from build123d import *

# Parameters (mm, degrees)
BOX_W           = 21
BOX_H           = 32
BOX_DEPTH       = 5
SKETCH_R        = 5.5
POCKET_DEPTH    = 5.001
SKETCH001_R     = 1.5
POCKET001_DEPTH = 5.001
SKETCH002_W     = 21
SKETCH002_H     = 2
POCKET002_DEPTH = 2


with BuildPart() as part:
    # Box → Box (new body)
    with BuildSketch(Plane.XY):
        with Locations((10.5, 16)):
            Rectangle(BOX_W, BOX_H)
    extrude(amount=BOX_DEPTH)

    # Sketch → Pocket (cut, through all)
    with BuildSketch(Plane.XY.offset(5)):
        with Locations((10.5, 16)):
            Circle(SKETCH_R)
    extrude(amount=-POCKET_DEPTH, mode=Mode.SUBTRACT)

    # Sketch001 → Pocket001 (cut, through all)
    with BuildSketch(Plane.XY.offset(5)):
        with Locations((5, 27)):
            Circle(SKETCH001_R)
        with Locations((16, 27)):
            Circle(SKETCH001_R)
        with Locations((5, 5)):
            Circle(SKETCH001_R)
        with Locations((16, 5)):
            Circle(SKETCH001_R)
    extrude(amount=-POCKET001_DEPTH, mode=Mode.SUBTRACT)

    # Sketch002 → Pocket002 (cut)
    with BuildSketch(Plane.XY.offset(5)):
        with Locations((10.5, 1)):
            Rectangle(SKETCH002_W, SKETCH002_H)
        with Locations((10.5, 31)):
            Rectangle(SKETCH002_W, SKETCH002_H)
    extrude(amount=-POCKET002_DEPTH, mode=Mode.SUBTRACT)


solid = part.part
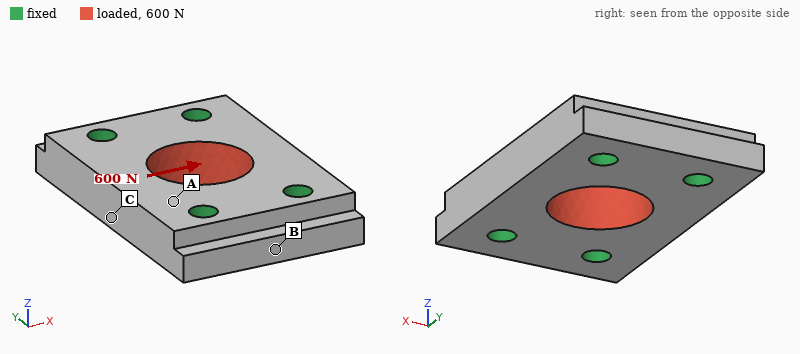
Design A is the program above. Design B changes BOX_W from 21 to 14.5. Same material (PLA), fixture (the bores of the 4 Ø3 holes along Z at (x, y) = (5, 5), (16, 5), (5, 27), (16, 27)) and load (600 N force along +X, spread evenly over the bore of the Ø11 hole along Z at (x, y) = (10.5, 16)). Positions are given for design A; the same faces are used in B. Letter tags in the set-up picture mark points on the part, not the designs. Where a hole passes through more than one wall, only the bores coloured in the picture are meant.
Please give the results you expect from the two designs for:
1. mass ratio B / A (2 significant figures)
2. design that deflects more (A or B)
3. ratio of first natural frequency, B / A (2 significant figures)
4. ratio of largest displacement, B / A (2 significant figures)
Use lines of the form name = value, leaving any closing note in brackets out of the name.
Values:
mass ratio B / A = 0.62
design that deflects more = B
ratio of first natural frequency, B / A = 1.2
ratio of largest displacement, B / A = 2.2
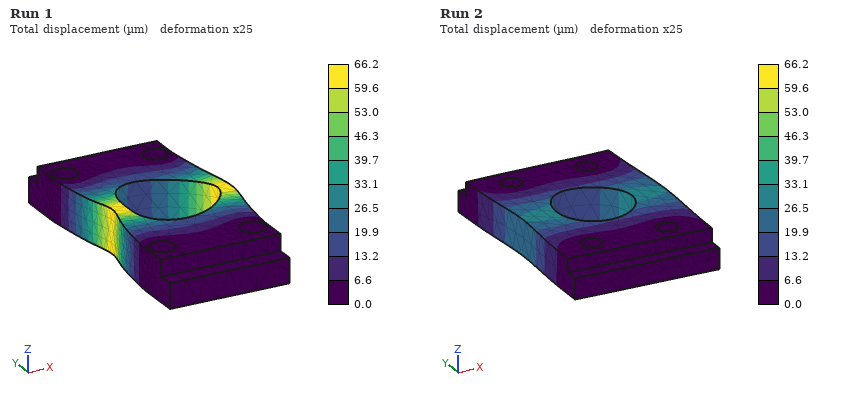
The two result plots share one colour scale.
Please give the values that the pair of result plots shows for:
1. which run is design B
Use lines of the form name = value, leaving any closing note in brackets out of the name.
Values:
which run is design B = Run 1
